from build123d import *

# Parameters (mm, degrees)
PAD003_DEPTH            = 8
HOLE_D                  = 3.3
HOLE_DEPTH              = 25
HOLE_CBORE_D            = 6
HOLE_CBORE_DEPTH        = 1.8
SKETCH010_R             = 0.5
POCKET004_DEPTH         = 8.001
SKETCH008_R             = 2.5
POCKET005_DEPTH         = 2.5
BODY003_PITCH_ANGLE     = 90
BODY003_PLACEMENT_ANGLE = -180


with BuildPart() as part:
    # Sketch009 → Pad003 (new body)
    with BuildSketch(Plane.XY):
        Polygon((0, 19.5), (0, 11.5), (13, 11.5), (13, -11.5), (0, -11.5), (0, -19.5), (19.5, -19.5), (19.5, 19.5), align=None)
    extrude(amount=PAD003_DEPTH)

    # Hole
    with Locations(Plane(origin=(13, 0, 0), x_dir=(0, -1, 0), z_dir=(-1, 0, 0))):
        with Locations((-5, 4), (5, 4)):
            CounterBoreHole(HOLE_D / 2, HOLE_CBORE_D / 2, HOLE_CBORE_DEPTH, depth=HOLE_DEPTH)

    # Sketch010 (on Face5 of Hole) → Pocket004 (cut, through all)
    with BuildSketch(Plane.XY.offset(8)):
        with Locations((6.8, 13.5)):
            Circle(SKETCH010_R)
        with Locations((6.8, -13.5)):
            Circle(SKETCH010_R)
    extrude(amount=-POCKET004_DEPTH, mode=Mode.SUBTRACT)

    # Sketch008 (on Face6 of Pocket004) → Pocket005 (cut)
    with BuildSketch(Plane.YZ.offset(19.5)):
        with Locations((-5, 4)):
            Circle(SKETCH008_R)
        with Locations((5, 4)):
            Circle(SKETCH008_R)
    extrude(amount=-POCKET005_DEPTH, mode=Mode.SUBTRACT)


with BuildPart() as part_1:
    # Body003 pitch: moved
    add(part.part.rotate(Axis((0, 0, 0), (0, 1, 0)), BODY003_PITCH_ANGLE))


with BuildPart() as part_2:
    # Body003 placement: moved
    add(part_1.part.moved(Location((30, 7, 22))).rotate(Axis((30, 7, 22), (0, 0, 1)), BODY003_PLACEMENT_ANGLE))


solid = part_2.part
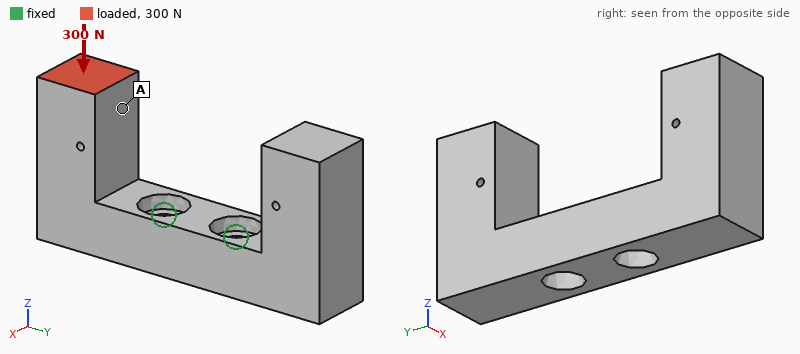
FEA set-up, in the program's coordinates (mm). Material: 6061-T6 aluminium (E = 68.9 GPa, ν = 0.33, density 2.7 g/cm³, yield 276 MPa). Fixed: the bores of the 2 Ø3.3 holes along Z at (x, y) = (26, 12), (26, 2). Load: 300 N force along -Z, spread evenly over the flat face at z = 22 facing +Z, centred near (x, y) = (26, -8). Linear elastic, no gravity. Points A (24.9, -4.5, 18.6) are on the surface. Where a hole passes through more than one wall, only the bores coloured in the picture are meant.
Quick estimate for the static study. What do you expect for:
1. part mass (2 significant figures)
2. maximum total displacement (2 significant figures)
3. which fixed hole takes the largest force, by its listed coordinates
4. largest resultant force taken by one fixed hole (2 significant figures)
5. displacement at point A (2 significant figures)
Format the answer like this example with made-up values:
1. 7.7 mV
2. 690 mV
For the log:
1. 9.3 g
2. 70 µm
3. (26, 2)
4. 480 N
5. 46 µm
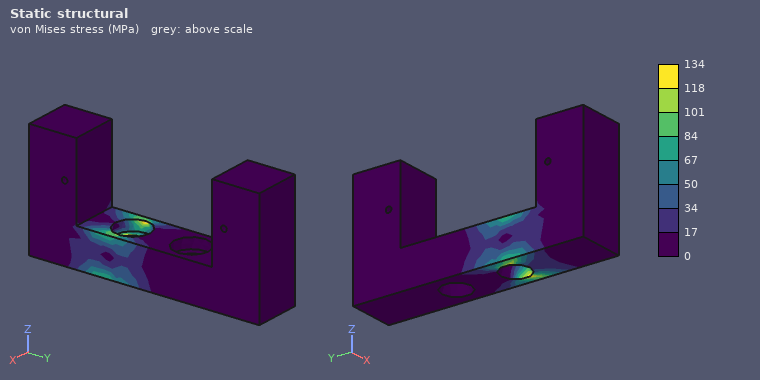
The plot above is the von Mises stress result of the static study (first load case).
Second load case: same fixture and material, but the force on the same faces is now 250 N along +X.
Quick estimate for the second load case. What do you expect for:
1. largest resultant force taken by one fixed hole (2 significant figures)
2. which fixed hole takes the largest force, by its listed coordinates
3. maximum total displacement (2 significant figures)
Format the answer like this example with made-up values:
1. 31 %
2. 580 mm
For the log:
1. 400 N
2. (26, 2)
3. 0.13 mm
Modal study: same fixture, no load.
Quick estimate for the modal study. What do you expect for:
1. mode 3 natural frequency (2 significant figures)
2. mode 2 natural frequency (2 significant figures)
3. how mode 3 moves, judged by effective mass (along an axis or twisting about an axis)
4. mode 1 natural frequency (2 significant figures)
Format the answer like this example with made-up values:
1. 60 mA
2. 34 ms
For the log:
1. 6800 Hz
2. 6000 Hz
3. along X
4. 5900 Hz
